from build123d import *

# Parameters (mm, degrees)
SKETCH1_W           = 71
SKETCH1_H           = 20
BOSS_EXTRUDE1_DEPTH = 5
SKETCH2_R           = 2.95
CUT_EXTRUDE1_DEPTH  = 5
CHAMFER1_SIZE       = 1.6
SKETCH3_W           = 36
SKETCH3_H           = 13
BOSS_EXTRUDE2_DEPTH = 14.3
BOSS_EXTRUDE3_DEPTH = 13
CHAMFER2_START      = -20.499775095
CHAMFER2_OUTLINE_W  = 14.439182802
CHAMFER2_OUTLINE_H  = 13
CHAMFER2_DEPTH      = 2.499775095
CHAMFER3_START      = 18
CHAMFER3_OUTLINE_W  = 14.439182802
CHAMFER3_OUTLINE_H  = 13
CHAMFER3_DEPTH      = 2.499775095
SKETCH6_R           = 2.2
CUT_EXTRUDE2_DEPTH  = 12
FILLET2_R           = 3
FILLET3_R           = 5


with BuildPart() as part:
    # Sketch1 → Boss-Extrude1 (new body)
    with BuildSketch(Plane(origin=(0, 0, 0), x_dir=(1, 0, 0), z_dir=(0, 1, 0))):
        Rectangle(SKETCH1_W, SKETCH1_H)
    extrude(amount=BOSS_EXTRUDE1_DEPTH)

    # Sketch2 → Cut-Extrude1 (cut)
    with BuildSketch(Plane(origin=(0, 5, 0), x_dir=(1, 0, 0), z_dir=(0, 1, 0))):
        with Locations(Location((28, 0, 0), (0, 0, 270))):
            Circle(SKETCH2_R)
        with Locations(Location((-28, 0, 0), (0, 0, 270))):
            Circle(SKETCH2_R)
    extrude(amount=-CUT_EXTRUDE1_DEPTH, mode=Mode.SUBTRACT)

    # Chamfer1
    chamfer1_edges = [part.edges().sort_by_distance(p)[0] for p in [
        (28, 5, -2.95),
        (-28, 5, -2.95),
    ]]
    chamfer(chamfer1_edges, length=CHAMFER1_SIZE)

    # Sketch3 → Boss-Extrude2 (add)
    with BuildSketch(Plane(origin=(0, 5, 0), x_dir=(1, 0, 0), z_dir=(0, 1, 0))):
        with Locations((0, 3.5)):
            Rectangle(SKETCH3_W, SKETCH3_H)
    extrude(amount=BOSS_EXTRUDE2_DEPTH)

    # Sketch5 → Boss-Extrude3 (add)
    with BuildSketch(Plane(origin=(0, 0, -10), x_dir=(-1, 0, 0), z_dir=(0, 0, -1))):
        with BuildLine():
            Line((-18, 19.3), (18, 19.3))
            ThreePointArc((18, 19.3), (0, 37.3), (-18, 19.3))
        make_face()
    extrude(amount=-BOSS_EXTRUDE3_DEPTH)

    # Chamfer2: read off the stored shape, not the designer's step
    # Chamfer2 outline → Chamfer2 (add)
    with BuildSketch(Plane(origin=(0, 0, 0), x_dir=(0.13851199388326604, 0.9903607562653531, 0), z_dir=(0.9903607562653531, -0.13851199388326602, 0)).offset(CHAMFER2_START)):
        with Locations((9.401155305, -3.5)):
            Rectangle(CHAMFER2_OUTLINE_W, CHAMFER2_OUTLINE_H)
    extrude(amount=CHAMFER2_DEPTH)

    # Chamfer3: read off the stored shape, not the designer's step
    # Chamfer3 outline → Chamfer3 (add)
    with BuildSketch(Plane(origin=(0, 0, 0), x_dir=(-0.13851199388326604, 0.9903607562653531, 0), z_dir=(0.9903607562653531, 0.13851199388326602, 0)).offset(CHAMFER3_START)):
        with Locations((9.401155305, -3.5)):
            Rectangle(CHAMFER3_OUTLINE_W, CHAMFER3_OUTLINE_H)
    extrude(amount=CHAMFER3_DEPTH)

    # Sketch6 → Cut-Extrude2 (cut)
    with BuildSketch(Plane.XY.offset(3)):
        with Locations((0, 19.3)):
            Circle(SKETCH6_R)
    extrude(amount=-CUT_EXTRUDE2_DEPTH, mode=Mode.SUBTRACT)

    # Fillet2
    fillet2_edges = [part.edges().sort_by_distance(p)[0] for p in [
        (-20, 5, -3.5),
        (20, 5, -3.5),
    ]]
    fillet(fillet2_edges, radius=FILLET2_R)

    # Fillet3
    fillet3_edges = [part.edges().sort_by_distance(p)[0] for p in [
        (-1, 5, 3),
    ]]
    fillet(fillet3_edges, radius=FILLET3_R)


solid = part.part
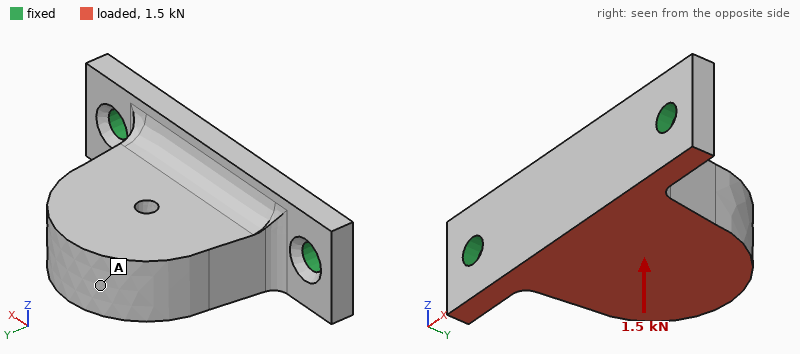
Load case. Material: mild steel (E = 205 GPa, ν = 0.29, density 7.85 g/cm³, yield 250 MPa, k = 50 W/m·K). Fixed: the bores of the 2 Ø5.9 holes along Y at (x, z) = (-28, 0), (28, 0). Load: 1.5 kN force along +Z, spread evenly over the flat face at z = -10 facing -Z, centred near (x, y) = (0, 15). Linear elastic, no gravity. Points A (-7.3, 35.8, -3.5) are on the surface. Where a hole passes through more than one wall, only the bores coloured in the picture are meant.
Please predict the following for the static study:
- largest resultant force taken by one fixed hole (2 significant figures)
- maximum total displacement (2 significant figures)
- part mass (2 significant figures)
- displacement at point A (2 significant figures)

750 N
57 µm
160 g
53 µm
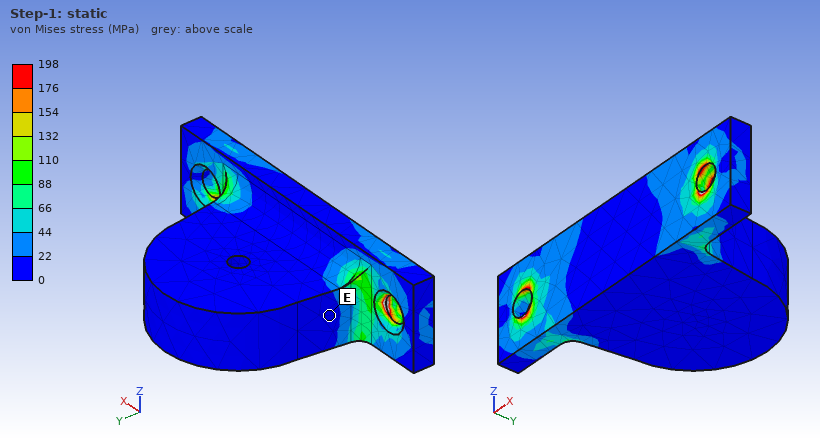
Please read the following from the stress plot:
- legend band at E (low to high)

0 to 22 MPa
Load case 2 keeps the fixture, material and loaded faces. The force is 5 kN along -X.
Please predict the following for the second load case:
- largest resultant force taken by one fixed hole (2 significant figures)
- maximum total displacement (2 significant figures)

3.0 kN
11 µm
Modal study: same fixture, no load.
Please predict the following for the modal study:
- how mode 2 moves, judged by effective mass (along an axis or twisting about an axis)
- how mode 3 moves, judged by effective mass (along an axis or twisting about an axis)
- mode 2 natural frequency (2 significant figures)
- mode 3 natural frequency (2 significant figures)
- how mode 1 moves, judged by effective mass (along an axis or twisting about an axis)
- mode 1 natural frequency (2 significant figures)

along Y
along X
9000 Hz
11 kHz
along Z
2700 Hz
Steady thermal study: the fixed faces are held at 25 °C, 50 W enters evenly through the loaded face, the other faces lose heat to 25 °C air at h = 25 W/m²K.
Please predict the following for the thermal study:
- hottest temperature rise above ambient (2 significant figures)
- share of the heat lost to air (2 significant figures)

78 K
12 %
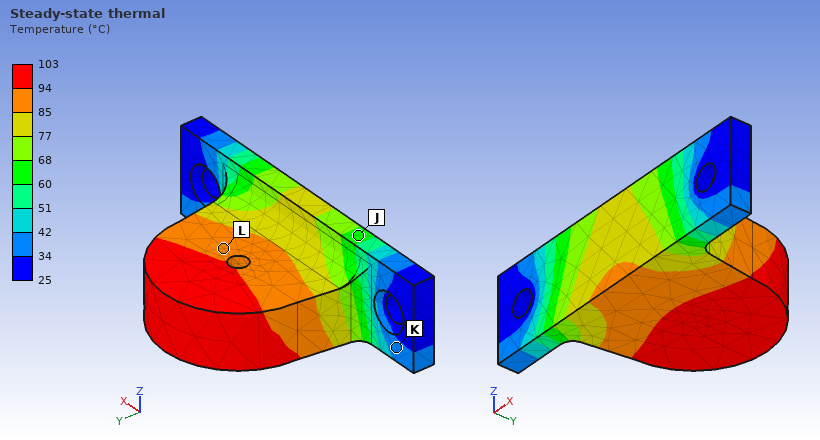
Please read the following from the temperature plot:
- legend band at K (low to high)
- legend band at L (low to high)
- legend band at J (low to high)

34 to 42 °C
85 to 94 °C
60 to 68 °C
